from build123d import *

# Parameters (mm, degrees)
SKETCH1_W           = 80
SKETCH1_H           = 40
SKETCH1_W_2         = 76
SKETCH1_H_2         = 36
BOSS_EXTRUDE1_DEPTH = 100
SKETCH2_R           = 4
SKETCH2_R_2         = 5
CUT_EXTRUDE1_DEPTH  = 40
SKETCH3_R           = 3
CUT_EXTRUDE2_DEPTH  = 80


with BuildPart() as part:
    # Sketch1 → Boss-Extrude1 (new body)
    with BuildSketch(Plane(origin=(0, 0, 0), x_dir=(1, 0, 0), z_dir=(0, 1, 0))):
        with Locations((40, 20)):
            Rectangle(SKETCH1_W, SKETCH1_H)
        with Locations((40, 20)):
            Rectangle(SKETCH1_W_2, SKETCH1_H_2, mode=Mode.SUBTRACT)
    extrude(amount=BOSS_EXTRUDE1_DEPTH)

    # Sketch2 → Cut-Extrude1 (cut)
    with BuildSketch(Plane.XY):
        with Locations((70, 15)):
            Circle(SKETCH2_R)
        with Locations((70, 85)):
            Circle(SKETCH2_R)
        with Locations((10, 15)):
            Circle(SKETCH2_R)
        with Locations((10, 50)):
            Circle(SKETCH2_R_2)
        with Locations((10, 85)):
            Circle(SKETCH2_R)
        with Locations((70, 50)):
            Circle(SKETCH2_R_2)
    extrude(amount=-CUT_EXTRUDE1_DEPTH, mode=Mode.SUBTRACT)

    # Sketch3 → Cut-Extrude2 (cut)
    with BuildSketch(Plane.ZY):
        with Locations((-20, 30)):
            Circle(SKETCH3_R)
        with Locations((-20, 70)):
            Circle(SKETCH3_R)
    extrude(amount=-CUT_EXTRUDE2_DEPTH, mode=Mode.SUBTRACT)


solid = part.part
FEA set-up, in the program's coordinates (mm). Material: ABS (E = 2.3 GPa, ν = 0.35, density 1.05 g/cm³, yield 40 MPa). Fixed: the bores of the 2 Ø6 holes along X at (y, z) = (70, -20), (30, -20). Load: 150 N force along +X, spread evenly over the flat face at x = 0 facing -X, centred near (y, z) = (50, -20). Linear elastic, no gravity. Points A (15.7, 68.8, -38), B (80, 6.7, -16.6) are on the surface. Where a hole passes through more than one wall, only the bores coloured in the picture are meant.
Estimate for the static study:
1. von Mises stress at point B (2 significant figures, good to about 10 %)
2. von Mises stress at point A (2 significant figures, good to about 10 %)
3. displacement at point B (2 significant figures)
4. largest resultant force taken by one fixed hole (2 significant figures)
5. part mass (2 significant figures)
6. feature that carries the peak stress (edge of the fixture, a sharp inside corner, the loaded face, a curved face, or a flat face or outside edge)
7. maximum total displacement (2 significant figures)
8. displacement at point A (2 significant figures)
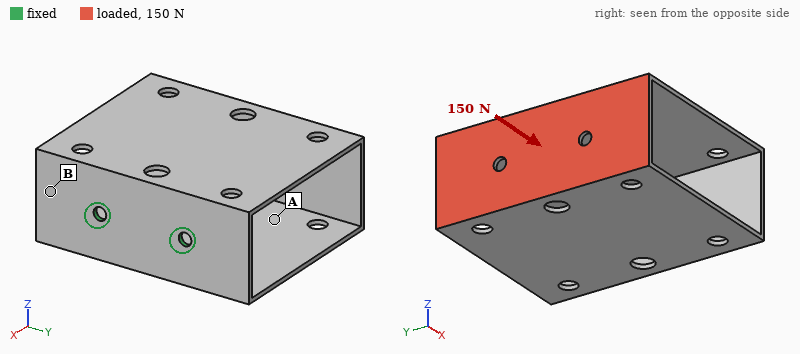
7.0 MPa
2.5 MPa
0.32 mm
75 N
47 g
a flat face or outside edge
1.3 mm
0.92 mm
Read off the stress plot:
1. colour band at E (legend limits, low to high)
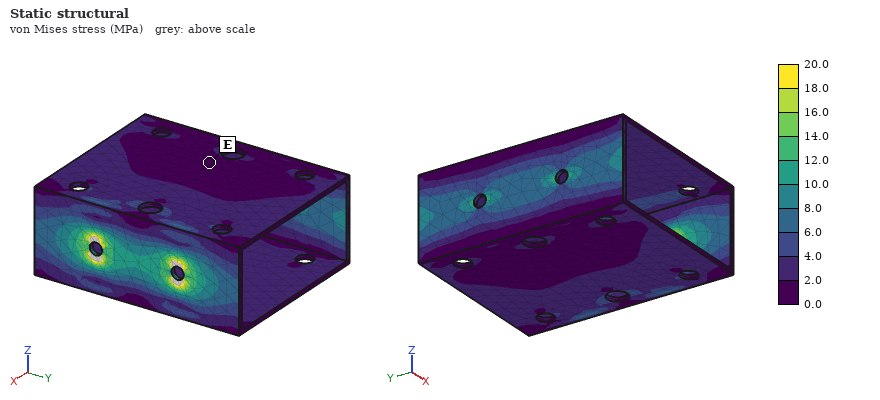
0.0 to 2.0 MPa
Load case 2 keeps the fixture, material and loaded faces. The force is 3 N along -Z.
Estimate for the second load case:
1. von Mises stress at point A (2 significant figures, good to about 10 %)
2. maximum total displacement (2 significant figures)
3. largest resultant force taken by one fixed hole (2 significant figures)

0.64 MPa
1.3 mm
1.5 N
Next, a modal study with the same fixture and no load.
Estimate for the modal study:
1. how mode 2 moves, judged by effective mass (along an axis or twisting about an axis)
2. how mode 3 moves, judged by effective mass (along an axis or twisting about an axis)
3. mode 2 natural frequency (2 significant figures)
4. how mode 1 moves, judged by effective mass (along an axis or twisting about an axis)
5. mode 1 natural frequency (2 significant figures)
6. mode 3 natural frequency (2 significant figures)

along Y
twisting about X
150 Hz
along Z
56 Hz
190 Hz
